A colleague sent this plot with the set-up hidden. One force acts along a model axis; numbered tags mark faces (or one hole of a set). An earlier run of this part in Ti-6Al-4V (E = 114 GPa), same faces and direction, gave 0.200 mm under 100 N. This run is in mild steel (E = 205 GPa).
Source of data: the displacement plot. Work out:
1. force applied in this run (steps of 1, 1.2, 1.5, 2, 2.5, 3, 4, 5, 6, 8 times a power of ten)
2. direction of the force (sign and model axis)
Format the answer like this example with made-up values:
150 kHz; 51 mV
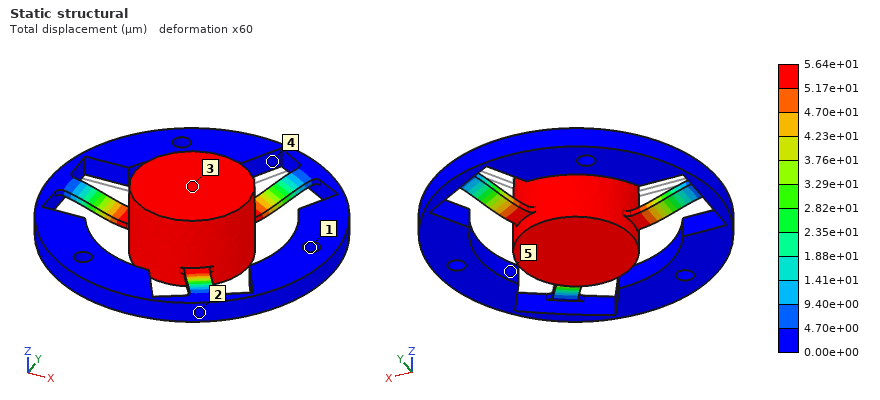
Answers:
50 N; -Z
